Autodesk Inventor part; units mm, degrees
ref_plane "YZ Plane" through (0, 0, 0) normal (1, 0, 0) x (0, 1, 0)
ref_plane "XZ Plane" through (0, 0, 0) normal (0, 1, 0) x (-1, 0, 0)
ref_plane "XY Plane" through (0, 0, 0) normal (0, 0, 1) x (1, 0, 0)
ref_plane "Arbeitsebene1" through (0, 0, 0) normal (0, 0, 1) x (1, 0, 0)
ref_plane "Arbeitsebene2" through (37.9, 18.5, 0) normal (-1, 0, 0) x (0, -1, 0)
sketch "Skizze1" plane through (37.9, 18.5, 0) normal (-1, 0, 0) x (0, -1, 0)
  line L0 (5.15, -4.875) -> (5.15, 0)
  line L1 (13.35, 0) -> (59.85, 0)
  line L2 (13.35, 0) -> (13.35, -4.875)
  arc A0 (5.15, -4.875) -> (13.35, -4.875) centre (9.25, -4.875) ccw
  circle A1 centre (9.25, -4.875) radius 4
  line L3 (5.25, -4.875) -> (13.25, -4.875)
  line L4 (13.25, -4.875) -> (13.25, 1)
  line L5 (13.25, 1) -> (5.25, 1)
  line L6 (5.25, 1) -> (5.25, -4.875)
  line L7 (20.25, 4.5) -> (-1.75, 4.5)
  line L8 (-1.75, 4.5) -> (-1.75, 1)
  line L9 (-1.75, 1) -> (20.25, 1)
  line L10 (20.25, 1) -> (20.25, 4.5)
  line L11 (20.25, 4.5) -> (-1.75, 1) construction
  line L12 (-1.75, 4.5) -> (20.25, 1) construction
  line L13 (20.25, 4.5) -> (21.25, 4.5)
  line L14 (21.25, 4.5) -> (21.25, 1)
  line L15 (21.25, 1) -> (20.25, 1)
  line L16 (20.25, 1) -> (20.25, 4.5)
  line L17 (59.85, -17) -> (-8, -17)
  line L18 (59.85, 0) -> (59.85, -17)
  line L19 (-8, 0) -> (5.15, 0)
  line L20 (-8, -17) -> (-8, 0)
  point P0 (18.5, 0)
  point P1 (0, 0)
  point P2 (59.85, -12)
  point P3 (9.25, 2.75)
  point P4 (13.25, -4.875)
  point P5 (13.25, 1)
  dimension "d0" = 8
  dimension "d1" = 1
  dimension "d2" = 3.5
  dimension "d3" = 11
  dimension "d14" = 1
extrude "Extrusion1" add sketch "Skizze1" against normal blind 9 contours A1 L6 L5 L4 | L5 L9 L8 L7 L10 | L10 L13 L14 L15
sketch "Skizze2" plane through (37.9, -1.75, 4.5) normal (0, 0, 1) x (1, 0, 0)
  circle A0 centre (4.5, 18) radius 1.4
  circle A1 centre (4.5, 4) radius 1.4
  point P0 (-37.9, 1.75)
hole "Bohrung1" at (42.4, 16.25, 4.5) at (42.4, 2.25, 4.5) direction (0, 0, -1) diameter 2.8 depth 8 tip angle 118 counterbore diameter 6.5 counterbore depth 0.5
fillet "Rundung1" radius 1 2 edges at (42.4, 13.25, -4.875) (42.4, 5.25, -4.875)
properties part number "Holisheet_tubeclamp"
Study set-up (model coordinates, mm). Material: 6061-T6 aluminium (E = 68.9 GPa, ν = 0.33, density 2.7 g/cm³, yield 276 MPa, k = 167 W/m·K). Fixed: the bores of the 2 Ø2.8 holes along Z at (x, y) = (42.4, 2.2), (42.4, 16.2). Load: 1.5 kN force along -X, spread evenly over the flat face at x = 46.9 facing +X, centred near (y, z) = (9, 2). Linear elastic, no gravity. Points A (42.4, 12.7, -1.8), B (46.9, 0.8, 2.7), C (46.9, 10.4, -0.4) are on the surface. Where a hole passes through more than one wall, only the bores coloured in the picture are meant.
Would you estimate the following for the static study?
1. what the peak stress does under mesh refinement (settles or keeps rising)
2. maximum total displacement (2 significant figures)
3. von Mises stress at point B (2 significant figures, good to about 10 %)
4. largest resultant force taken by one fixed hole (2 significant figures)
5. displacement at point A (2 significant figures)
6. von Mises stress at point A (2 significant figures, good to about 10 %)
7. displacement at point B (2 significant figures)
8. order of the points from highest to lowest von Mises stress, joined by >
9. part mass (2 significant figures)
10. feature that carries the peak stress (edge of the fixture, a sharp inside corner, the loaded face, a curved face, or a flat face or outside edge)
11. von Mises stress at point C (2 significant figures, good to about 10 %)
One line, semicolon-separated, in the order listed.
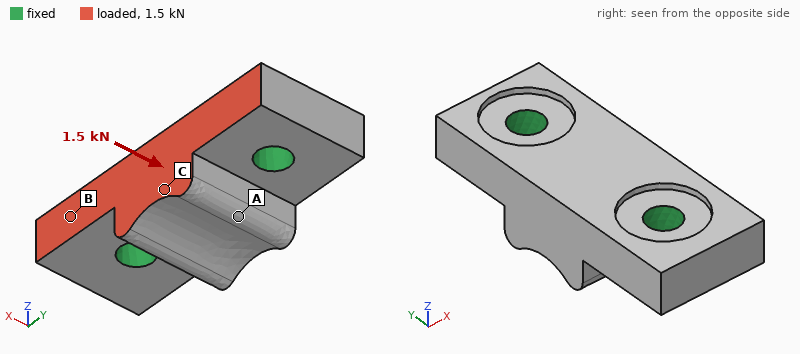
keeps rising; 6.2 µm; 25 MPa; 790 N; 4.8 µm; 8.3 MPa; 1.2 µm; B > C > A; 2.2 g; edge of the fixture; 13 MPa
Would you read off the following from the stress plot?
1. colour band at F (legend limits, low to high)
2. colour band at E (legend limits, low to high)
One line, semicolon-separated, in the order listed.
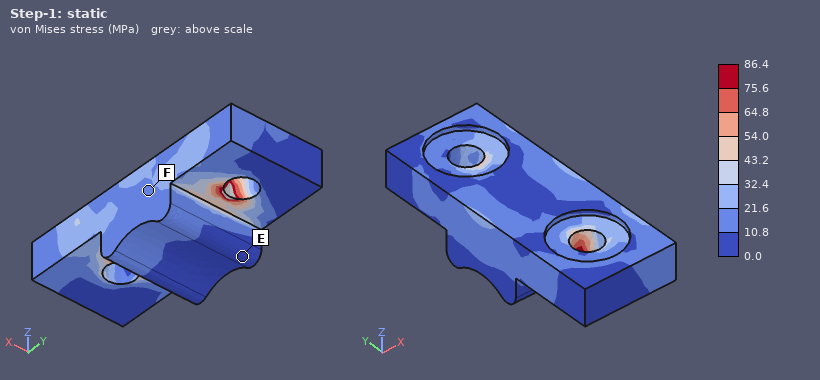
10.8 to 21.6 MPa; 0.0 to 10.8 MPa
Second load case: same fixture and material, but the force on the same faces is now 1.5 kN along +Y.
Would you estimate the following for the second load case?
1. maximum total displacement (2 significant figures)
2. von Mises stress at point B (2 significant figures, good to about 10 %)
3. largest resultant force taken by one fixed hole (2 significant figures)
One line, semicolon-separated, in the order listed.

7.2 µm; 34 MPa; 870 N
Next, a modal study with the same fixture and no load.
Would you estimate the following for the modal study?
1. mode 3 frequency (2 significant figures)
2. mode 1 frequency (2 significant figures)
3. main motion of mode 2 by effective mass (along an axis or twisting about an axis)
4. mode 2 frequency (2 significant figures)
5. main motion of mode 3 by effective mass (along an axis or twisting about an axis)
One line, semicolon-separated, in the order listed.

77 kHz; 50 kHz; along Z; 63 kHz; along X
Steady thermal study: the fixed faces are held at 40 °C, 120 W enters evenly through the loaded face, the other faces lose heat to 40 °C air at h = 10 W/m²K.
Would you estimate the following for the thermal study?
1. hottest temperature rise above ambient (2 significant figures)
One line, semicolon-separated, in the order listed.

56 K
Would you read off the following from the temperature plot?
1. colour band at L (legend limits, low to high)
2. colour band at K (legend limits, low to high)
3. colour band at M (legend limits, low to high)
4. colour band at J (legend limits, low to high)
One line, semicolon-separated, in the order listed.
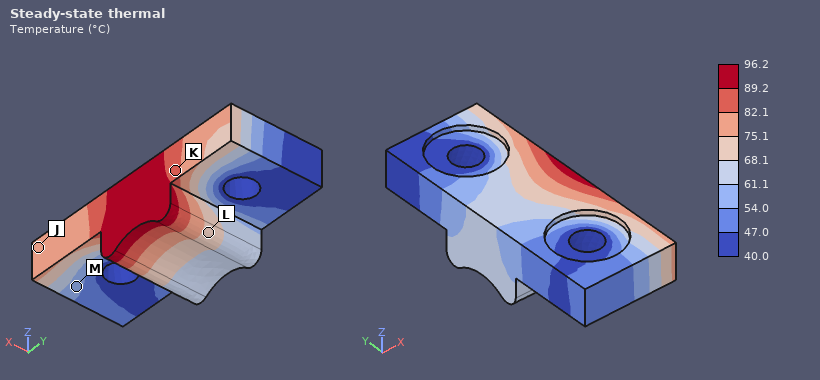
68.1 to 75.1 °C; 82.1 to 89.2 °C; 54.0 to 61.1 °C; 75.1 to 82.1 °C
